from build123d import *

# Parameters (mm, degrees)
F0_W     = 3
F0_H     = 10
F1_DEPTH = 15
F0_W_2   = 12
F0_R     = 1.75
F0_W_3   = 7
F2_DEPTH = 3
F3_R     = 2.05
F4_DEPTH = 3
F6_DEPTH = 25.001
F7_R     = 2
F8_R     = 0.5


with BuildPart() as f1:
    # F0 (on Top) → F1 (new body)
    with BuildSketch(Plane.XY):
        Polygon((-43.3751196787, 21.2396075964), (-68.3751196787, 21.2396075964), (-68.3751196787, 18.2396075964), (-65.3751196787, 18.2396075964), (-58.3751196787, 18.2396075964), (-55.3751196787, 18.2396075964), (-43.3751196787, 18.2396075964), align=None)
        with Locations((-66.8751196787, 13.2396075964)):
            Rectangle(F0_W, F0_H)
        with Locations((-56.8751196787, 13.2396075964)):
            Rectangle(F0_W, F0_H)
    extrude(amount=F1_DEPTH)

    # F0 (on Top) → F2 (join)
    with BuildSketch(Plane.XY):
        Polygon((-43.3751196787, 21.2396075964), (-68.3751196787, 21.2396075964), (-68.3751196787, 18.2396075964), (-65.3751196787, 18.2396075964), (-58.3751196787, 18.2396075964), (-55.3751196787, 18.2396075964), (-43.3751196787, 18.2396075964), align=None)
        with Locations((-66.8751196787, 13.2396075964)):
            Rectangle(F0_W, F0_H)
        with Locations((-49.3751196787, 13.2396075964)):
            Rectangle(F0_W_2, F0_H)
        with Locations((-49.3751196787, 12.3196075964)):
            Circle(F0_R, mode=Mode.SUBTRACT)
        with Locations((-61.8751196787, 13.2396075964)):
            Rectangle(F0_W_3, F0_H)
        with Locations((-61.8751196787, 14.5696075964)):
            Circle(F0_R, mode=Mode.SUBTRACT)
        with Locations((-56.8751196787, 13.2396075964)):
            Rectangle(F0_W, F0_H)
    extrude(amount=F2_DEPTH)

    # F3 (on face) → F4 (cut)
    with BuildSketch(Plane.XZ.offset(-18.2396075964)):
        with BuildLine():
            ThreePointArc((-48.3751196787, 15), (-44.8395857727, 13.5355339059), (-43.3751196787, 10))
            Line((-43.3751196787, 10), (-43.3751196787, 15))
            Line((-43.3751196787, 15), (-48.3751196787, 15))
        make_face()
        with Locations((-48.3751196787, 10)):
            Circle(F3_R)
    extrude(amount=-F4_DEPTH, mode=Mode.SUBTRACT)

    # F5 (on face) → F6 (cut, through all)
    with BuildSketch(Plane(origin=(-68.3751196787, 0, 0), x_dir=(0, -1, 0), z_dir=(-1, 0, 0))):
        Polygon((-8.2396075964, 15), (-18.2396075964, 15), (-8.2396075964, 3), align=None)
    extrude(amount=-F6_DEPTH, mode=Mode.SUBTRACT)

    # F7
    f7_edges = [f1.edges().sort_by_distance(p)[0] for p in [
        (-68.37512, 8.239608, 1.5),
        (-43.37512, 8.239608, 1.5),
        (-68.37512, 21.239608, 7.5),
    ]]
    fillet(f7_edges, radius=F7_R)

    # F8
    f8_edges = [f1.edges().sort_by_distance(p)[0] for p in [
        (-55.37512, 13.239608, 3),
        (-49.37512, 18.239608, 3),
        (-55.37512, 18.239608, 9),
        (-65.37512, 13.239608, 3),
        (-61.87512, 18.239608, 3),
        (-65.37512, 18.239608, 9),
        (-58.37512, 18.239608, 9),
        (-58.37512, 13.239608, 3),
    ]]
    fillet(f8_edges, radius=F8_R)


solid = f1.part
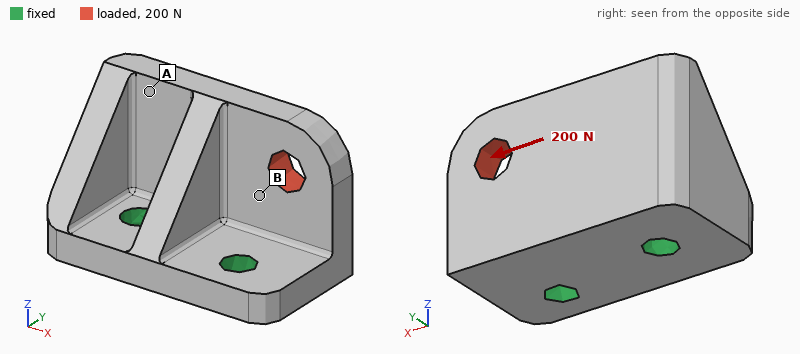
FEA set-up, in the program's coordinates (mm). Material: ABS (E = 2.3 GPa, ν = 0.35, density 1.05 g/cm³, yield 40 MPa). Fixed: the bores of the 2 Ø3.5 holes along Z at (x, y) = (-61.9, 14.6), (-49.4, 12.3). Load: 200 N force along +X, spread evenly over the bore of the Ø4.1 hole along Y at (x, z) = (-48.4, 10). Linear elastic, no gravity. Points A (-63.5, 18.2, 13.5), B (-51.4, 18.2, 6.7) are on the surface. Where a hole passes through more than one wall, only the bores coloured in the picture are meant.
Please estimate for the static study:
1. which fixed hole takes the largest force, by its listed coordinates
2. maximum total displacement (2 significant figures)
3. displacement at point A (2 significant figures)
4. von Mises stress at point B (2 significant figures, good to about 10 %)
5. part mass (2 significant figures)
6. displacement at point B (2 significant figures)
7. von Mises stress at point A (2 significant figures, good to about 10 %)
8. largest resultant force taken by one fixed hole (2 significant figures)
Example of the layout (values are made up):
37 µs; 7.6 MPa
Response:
(-61.9, 14.6); 0.23 mm; 0.15 mm; 11 MPa; 2.2 g; 0.10 mm; 4.7 MPa; 180 N
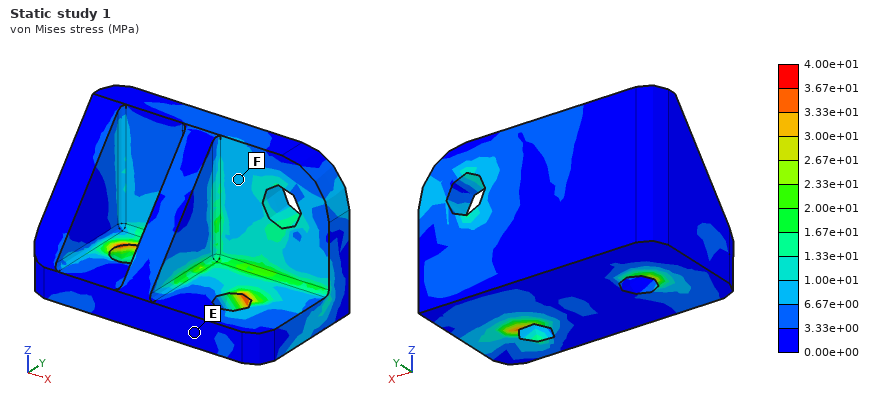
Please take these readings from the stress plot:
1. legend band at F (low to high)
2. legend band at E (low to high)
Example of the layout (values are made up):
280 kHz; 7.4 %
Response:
6.67e+00 to 1.00e+01 MPa; 0.00e+00 to 3.33e+00 MPa
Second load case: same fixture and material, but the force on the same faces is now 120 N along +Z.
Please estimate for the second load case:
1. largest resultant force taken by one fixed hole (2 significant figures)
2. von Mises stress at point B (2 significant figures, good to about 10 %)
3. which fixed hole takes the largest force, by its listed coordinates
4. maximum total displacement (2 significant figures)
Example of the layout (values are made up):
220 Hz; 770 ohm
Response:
110 N; 6.2 MPa; (-49.4, 12.3); 0.28 mm
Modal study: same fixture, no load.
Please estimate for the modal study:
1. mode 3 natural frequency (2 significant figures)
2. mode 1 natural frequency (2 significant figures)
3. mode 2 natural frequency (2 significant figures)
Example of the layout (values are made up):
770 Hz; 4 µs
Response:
7400 Hz; 3900 Hz; 5300 Hz
